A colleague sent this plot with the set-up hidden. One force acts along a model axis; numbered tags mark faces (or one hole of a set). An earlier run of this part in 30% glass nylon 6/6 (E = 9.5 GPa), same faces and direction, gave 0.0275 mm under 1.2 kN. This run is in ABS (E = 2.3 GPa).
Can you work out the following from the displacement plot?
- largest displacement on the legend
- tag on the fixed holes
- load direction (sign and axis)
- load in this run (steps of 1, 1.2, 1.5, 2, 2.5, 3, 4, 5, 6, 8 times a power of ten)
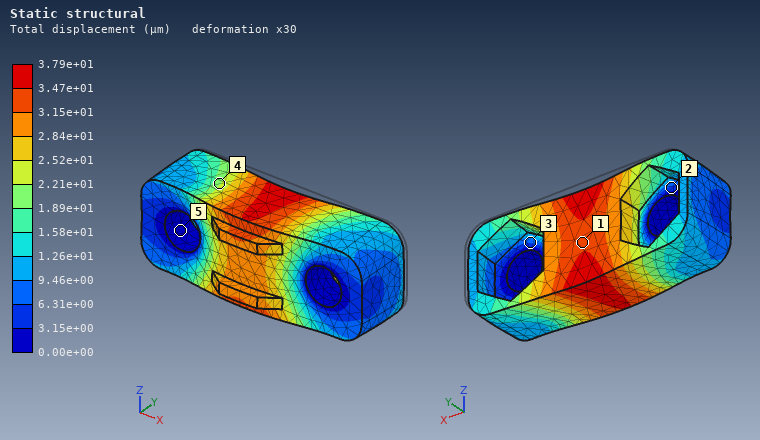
3.79e+01 µm
5
-Y
400 N
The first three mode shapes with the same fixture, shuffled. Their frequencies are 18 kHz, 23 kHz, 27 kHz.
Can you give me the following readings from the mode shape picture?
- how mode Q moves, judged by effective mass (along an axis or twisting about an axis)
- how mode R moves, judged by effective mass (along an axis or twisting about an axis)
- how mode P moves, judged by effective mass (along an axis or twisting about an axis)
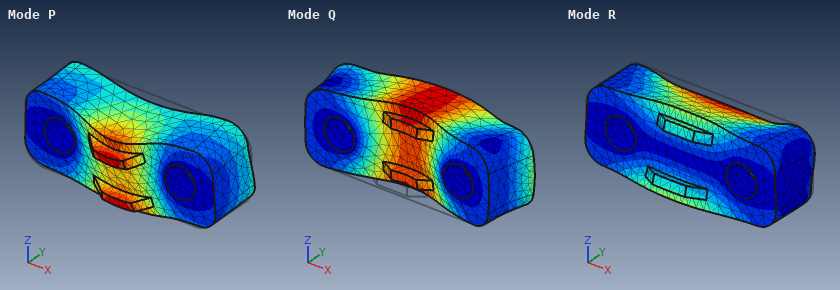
along Y
along Z
along Z
